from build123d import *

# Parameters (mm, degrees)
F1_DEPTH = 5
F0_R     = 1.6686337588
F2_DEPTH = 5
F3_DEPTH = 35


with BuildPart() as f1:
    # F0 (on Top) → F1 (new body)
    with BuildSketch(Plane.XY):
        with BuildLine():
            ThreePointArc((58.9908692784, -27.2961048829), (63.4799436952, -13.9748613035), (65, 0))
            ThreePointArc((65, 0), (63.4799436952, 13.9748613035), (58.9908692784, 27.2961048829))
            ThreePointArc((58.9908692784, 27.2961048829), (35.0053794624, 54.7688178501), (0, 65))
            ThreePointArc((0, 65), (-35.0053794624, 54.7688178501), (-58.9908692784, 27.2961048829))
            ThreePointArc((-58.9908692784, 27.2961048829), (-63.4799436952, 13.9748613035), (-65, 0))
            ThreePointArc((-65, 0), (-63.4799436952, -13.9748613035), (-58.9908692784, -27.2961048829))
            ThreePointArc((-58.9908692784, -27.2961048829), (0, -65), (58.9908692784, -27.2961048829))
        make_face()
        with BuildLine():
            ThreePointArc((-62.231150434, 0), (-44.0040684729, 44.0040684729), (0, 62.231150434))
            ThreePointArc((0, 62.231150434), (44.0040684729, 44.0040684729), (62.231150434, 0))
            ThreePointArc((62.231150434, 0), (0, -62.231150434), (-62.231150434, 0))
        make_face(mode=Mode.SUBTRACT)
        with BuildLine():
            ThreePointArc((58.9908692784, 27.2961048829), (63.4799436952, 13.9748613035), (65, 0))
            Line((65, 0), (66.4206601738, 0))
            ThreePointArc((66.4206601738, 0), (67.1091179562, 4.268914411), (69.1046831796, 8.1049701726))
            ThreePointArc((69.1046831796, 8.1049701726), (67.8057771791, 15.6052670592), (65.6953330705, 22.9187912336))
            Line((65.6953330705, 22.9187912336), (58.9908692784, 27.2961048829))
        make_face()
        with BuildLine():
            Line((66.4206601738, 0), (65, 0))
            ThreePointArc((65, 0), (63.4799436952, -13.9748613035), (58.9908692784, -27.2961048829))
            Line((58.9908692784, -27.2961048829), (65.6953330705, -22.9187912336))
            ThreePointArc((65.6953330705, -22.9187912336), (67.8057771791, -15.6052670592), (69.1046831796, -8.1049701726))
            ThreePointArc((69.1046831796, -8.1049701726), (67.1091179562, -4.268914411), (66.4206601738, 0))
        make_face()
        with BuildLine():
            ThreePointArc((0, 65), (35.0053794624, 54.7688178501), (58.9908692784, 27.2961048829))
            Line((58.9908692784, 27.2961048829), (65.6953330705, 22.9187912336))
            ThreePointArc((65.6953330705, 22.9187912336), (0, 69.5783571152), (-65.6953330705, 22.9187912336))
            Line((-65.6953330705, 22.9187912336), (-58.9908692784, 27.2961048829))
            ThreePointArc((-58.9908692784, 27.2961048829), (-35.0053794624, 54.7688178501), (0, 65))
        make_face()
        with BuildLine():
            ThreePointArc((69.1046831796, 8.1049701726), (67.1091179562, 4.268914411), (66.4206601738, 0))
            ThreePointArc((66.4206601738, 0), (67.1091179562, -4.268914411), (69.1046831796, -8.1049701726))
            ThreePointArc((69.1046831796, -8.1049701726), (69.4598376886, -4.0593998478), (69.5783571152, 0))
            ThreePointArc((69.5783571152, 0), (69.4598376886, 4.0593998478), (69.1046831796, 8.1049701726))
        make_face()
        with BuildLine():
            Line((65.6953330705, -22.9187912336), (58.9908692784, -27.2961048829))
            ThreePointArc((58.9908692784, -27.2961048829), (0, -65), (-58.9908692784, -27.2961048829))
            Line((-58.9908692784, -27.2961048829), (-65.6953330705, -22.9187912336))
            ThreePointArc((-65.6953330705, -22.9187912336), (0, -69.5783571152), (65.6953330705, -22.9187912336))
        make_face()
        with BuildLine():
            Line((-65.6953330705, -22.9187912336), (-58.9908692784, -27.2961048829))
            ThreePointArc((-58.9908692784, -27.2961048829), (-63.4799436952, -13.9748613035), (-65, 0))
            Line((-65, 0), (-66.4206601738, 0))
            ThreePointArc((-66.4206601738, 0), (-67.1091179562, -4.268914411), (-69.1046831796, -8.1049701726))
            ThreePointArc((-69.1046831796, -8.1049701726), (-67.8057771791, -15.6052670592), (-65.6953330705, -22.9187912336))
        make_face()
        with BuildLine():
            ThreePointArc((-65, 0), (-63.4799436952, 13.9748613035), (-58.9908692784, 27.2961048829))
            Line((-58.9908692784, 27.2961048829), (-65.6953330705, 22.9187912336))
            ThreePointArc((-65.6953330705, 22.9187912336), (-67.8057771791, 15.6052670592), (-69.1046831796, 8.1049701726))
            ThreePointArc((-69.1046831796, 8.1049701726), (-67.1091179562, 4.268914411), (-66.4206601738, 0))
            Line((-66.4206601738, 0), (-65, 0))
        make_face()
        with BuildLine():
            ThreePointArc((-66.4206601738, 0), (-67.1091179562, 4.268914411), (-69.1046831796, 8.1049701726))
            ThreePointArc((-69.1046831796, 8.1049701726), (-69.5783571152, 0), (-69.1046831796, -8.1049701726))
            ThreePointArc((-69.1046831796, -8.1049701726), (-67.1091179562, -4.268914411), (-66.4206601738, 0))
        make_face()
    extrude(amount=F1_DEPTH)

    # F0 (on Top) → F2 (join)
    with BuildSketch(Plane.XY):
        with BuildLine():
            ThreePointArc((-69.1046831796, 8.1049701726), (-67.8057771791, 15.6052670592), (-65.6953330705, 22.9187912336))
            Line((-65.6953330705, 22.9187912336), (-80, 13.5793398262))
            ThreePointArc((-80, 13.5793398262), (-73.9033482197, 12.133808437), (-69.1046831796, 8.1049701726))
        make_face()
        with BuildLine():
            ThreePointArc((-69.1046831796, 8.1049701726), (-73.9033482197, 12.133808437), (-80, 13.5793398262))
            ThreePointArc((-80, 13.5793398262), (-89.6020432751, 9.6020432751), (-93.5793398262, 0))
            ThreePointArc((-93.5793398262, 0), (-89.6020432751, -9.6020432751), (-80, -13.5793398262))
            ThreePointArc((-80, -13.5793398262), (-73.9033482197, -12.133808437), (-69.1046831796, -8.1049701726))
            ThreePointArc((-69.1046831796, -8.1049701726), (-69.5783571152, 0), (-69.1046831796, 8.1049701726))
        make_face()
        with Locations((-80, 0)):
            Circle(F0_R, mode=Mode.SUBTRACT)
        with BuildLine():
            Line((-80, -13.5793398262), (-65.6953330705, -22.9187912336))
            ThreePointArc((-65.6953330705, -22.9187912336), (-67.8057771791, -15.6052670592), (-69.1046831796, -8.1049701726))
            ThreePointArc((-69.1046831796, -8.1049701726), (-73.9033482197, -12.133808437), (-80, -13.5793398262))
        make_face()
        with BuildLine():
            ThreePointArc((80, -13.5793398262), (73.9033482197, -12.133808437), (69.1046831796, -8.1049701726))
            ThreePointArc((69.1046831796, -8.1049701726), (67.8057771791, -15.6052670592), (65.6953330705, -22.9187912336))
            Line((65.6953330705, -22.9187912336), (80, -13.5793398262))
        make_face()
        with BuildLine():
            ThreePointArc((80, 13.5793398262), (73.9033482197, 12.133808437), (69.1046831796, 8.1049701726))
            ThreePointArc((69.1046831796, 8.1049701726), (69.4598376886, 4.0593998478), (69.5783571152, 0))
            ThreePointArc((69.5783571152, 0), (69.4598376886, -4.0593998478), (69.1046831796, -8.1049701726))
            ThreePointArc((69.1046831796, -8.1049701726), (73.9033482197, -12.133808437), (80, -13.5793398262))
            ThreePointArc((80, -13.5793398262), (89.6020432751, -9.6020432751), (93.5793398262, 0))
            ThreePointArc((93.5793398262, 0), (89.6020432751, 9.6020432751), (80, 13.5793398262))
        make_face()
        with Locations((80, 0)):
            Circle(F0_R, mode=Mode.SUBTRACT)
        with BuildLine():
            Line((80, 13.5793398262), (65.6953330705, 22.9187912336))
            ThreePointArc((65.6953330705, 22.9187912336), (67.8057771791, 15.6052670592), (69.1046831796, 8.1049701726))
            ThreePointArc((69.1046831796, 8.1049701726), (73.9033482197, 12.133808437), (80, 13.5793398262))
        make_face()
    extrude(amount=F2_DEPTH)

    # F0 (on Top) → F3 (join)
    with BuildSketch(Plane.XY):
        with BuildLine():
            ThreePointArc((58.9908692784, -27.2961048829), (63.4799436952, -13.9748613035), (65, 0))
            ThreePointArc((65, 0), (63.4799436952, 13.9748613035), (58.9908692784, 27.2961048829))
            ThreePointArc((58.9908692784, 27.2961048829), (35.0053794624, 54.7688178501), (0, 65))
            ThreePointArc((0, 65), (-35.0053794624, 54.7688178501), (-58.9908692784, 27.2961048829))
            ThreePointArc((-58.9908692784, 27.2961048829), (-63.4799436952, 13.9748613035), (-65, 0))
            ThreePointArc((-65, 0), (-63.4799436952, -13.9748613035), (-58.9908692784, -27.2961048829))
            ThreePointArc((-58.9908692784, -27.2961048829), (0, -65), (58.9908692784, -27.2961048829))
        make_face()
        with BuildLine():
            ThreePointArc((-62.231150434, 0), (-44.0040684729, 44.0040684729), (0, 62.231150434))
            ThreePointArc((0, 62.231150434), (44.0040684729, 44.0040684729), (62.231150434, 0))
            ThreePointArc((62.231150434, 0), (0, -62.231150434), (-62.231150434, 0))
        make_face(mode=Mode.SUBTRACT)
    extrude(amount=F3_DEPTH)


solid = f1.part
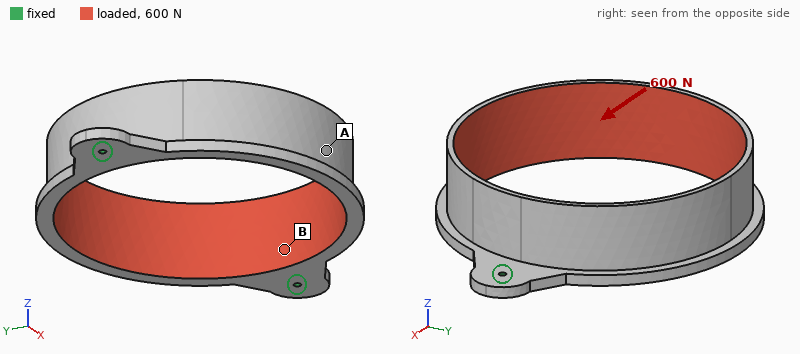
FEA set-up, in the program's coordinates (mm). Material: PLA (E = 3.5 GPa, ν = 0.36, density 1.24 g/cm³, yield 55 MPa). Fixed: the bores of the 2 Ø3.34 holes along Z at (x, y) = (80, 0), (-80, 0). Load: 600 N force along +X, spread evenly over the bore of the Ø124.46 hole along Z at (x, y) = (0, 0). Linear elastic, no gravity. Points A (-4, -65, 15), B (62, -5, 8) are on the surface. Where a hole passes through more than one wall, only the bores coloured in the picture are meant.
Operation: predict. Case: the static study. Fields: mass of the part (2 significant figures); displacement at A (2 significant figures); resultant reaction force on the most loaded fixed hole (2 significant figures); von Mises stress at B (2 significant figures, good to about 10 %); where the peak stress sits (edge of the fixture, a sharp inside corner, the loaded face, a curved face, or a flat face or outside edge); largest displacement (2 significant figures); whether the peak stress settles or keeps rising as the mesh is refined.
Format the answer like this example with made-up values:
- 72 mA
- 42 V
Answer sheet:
- 69 g
- 0.55 mm
- 310 N
- 4.8 MPa
- a sharp inside corner
- 0.77 mm
- keeps rising
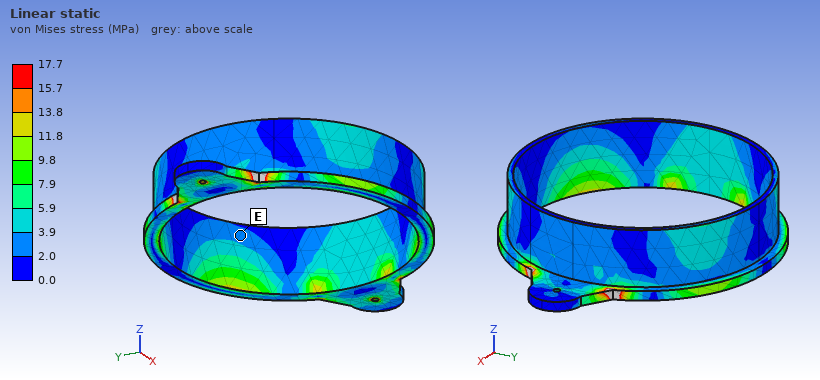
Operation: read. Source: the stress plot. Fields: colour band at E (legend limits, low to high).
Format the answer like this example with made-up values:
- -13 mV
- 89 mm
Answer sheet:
- 2.0 to 3.9 MPa
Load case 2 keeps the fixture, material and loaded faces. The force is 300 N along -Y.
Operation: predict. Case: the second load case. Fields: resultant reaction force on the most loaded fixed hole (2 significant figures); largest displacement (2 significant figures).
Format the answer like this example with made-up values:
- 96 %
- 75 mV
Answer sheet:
- 150 N
- 2.5 mm
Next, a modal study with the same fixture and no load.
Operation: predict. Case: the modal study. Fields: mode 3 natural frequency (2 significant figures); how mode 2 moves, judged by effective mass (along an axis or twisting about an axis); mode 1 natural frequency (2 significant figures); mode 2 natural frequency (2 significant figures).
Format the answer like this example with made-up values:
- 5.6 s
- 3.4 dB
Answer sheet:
- 360 Hz
- along Z
- 160 Hz
- 250 Hz
